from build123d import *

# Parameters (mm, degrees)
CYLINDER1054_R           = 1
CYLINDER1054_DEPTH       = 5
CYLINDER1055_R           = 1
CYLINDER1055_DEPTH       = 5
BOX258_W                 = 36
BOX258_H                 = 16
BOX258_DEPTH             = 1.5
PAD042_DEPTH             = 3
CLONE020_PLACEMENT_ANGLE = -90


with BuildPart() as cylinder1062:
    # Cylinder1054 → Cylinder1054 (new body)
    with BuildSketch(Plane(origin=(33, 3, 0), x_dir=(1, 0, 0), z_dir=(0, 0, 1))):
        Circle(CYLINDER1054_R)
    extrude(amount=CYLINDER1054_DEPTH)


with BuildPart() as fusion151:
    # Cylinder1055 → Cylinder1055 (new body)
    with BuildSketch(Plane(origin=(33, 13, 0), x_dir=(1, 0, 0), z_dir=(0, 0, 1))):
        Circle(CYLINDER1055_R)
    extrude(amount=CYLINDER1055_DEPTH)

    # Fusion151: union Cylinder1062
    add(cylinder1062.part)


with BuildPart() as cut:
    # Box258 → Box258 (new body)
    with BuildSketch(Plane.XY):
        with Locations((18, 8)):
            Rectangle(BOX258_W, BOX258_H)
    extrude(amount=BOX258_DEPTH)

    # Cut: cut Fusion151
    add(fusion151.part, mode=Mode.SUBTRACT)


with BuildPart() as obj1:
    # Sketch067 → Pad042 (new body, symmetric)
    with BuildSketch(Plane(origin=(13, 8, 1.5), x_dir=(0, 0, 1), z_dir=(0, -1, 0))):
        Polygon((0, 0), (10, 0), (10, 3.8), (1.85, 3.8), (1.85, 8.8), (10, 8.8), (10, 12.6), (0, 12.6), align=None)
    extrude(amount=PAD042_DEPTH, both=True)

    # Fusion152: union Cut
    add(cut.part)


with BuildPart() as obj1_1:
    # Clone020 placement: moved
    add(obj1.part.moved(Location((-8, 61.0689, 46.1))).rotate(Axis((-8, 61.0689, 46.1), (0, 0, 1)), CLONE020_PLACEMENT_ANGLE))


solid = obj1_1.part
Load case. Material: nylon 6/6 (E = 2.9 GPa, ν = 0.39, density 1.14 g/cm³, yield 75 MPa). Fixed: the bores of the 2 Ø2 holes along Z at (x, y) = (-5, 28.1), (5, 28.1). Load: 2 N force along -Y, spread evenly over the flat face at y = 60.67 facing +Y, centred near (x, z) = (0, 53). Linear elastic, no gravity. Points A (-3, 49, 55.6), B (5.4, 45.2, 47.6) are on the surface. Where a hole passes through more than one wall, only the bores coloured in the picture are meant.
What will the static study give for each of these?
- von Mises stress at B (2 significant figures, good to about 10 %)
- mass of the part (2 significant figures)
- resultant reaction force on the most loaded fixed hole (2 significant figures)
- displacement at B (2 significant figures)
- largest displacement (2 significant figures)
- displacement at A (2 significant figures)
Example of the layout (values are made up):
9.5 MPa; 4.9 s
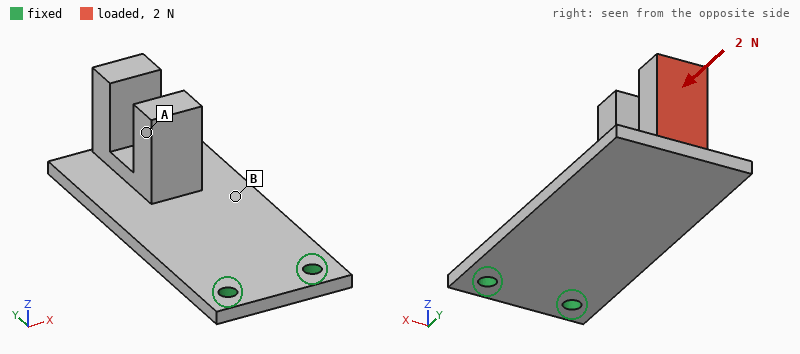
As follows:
1.8 MPa; 1.6 g; 1.0 N; 0.12 mm; 0.44 mm; 0.24 mm
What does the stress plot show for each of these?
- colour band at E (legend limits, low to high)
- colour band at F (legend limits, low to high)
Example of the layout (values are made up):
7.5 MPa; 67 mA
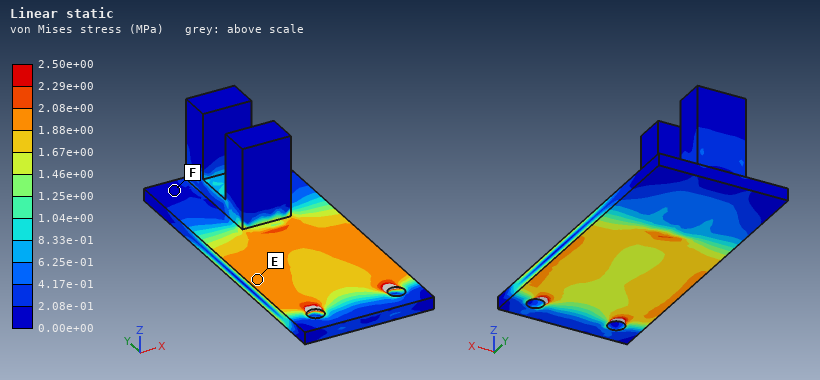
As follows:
1.88e+00 to 2.08e+00 MPa; 0.00e+00 to 2.08e-01 MPa
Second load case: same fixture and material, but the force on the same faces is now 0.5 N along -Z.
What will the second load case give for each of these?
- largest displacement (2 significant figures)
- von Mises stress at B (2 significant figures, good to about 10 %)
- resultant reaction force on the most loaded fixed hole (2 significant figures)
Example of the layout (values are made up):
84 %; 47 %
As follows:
0.44 mm; 1.2 MPa; 0.25 N
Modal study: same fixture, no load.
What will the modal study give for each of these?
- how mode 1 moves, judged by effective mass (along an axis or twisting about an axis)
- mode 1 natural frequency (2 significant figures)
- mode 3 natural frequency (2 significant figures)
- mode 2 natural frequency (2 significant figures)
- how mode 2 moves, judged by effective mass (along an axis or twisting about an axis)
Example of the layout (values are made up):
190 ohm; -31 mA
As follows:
along Z; 230 Hz; 1500 Hz; 900 Hz; along X
